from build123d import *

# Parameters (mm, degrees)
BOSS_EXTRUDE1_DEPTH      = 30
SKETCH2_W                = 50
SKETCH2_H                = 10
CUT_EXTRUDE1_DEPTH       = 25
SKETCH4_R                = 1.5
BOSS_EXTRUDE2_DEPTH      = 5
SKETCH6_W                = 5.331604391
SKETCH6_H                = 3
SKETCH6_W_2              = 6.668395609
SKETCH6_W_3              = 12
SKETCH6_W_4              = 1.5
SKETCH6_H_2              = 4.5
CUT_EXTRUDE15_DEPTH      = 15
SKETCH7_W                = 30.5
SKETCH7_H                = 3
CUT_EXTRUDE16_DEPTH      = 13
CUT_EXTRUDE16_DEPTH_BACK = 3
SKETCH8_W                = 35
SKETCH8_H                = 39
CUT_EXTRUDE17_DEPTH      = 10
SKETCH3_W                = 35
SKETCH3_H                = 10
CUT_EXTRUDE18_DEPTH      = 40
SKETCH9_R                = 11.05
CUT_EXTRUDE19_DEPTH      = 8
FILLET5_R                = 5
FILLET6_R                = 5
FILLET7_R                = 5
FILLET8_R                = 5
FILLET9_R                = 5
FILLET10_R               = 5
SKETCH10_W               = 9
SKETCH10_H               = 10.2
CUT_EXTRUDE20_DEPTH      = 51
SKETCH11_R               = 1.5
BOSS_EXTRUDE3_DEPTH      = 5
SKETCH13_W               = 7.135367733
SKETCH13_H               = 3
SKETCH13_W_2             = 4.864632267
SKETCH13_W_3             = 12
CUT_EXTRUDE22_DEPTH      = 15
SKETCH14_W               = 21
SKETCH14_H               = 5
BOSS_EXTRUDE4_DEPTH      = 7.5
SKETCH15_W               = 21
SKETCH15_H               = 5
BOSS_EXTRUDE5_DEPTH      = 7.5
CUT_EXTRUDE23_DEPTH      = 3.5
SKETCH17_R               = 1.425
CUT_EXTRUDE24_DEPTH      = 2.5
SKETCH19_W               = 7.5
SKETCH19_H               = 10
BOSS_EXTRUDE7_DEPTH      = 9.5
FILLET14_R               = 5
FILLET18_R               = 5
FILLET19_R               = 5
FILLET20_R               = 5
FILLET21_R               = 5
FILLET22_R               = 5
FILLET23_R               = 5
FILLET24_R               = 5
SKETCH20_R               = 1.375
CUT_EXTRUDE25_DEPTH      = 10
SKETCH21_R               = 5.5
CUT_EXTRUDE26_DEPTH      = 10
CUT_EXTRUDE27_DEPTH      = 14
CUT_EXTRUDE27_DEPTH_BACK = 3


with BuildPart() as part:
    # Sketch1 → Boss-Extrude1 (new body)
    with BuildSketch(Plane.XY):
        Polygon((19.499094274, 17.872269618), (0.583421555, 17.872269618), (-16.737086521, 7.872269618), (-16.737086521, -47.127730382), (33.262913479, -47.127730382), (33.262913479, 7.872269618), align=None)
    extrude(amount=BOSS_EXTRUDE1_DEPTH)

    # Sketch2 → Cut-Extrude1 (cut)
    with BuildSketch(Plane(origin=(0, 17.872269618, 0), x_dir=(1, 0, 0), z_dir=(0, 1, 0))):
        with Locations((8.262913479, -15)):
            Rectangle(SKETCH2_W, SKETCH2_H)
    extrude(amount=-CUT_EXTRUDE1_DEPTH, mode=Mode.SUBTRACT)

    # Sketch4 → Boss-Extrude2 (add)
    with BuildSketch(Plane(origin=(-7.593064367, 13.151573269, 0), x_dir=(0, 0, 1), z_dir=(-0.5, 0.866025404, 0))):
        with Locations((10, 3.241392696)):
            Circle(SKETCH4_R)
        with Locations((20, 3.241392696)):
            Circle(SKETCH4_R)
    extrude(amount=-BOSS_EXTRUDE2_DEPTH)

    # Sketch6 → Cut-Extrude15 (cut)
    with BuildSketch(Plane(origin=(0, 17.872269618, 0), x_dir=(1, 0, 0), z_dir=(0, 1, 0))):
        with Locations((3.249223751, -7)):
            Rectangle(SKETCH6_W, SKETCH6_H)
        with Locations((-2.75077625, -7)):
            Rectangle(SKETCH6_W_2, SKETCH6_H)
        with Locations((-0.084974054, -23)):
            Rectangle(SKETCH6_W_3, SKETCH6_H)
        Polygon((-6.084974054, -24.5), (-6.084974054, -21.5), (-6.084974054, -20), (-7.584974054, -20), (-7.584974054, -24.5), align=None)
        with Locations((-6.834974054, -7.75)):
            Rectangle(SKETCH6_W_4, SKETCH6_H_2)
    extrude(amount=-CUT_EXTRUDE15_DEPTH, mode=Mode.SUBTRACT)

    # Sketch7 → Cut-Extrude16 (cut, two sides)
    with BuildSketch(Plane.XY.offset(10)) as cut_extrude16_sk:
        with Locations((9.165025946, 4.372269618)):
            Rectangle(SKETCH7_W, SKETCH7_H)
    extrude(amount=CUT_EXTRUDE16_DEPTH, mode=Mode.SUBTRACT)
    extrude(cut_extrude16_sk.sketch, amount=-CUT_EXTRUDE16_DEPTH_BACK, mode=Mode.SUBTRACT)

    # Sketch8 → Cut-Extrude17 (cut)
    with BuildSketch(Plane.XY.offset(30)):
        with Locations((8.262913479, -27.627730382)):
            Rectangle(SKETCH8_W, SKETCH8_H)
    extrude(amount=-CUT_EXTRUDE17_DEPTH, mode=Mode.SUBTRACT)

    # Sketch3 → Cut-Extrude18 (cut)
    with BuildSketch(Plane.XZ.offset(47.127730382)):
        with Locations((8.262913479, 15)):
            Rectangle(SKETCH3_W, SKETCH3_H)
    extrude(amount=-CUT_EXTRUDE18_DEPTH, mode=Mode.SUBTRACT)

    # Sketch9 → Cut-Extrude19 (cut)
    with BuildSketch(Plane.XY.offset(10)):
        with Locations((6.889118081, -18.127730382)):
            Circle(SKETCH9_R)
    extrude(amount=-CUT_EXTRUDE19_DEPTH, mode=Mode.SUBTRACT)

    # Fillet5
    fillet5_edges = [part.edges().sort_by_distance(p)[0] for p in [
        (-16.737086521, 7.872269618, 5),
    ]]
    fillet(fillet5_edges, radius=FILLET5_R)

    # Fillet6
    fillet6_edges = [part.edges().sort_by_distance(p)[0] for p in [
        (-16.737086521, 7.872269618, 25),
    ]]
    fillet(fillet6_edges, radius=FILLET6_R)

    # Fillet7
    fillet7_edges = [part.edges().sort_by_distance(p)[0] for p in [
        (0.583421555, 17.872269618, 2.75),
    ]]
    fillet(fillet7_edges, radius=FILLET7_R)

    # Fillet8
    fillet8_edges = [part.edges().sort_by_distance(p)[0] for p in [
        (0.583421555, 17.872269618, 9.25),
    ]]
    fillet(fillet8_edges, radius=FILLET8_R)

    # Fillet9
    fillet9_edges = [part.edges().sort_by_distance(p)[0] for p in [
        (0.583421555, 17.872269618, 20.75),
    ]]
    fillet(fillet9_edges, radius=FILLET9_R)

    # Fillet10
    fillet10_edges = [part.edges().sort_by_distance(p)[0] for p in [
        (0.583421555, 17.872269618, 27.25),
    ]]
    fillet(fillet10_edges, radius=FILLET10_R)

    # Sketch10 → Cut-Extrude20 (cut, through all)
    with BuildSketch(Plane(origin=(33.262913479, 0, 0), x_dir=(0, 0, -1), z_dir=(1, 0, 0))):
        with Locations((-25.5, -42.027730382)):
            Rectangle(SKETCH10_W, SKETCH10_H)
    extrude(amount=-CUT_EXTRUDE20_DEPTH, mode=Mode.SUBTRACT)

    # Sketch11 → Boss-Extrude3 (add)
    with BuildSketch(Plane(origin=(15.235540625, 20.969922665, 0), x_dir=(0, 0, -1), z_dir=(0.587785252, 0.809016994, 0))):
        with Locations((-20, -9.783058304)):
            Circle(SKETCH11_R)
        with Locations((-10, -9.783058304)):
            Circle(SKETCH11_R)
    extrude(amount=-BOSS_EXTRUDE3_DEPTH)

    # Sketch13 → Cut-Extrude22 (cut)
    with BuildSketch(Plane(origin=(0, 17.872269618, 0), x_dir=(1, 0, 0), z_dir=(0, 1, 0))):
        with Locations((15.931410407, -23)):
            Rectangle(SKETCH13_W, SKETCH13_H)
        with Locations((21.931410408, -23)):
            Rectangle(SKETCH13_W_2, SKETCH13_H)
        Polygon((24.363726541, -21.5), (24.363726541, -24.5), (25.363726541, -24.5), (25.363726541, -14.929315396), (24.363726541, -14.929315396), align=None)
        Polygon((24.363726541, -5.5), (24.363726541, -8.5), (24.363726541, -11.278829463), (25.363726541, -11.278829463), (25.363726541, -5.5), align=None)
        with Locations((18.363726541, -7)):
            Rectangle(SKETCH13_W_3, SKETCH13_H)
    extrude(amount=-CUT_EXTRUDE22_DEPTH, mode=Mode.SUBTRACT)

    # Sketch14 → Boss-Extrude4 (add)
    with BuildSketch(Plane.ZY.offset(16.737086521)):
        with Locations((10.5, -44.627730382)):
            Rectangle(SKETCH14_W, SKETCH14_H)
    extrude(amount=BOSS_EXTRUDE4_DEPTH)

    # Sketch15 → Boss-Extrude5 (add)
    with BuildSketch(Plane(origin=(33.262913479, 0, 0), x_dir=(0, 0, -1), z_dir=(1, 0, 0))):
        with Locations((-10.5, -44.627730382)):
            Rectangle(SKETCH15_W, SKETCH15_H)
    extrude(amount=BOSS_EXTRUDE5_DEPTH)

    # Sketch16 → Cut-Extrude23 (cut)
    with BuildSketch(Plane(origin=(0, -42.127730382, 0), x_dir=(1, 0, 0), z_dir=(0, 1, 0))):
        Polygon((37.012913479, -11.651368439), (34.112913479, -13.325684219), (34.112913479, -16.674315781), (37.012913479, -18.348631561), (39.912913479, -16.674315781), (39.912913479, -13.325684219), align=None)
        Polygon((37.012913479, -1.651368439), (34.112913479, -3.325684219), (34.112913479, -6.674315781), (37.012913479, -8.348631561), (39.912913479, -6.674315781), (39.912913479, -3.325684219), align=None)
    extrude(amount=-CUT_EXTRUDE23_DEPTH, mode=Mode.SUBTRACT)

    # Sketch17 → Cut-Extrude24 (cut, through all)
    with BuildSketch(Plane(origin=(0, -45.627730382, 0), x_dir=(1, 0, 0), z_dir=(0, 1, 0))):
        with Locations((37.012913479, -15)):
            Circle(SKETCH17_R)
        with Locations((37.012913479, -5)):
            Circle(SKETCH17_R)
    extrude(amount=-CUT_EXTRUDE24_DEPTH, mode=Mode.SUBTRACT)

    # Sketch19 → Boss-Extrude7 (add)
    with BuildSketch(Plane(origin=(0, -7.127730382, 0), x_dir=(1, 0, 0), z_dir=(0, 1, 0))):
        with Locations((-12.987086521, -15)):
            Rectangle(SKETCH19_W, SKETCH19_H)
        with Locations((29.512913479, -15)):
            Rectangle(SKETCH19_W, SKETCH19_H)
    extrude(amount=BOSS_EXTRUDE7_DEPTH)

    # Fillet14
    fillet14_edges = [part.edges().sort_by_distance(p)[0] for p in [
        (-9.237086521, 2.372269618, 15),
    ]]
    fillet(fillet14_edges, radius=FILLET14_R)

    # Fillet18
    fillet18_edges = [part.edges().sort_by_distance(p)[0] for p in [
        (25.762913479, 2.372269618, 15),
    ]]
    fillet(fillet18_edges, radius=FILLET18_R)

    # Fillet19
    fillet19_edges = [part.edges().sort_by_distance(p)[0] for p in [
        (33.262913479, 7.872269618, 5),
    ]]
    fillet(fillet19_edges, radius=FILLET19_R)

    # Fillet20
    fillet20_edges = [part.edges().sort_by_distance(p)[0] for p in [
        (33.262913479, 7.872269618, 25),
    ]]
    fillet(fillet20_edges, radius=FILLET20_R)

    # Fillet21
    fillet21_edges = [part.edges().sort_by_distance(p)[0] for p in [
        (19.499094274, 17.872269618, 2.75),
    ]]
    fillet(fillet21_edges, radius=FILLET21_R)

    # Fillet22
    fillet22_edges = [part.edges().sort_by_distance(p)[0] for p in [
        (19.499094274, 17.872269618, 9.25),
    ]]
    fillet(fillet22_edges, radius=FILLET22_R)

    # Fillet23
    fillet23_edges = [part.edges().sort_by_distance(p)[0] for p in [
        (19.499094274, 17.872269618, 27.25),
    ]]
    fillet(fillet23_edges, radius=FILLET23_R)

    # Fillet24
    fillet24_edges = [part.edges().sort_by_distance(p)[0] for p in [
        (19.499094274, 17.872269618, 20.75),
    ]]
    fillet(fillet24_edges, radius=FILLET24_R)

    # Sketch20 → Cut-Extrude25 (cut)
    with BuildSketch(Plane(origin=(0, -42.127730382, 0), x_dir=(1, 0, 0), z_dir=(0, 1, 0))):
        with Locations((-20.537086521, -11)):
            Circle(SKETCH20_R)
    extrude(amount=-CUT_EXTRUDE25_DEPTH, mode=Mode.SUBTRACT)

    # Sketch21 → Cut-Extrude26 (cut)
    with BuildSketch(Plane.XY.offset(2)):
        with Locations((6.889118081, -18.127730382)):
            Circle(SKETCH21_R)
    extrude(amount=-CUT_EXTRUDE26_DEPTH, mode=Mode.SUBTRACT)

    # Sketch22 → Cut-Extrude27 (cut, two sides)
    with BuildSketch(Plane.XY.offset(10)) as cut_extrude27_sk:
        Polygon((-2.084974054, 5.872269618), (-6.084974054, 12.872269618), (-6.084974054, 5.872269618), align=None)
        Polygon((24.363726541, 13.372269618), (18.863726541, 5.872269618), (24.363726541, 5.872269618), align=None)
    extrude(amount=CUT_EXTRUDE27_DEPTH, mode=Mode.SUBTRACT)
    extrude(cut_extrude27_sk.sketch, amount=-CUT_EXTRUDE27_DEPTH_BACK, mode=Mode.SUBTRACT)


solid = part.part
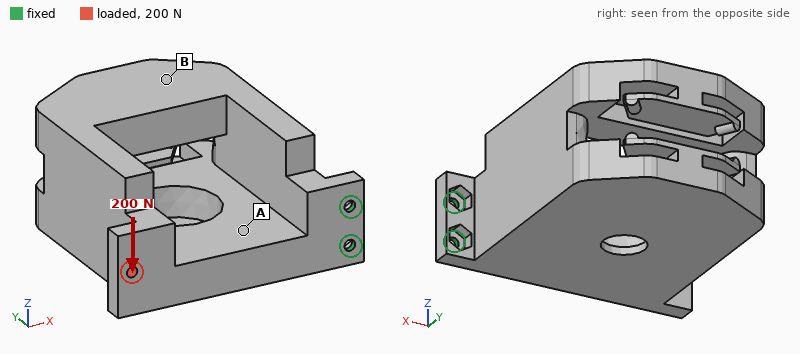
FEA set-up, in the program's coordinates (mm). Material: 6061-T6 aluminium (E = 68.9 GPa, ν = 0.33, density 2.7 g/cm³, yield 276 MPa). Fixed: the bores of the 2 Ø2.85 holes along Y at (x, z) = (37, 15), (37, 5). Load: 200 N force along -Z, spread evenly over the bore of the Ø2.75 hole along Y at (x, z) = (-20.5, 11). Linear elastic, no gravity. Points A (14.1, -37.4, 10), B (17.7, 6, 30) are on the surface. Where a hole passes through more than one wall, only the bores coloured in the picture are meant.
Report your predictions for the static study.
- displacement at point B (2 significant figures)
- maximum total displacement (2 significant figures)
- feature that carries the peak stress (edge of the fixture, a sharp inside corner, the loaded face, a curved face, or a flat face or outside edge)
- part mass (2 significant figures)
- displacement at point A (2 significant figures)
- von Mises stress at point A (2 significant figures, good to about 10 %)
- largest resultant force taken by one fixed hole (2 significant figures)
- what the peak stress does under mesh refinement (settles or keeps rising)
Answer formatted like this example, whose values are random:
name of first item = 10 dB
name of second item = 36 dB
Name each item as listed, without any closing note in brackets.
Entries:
displacement at point B = 0.044 mm
maximum total displacement = 0.16 mm
feature that carries the peak stress = edge of the fixture
part mass = 130 g
displacement at point A = 0.037 mm
von Mises stress at point A = 12 MPa
largest resultant force taken by one fixed hole = 970 N
what the peak stress does under mesh refinement = keeps rising
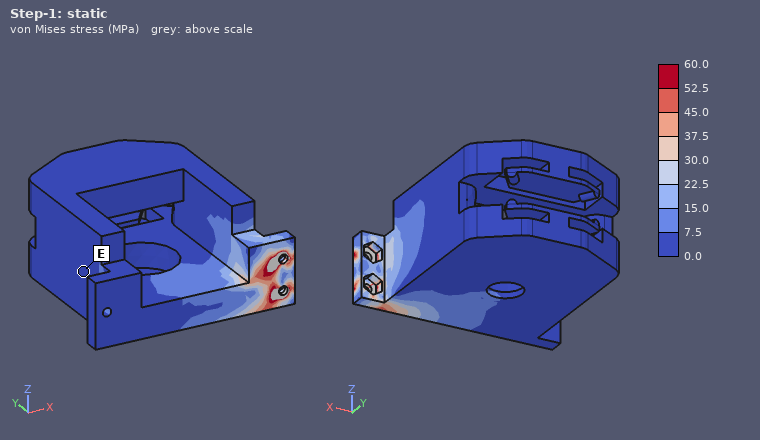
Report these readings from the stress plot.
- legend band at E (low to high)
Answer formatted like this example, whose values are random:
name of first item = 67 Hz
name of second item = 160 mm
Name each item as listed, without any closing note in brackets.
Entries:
legend band at E = 0.0 to 7.5 MPa
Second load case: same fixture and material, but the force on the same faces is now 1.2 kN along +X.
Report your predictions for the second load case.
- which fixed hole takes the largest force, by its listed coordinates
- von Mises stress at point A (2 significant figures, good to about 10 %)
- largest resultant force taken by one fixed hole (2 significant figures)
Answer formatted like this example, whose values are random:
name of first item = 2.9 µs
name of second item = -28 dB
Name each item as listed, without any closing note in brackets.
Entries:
which fixed hole takes the largest force, by its listed coordinates = (37, 15)
von Mises stress at point A = 18 MPa
largest resultant force taken by one fixed hole = 700 N
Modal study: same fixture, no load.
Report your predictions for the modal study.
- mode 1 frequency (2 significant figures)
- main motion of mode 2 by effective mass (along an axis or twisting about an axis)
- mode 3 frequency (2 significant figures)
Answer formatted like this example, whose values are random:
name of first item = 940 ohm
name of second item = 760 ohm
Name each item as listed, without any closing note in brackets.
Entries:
mode 1 frequency = 220 Hz
main motion of mode 2 by effective mass = along Z
mode 3 frequency = 1200 Hz
